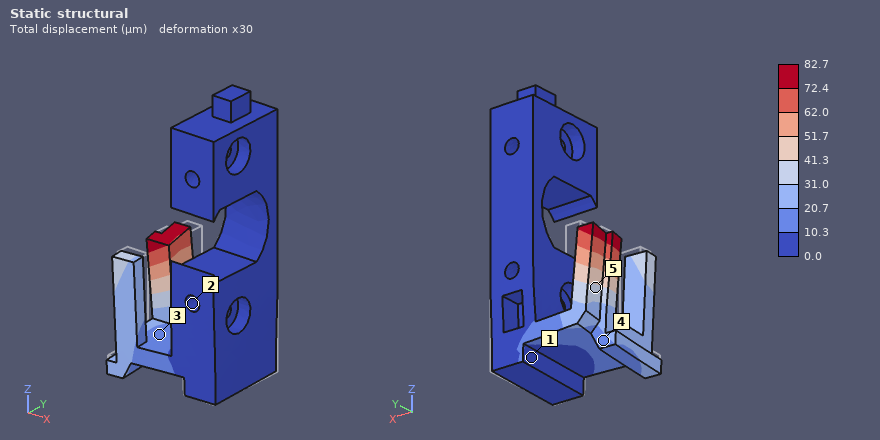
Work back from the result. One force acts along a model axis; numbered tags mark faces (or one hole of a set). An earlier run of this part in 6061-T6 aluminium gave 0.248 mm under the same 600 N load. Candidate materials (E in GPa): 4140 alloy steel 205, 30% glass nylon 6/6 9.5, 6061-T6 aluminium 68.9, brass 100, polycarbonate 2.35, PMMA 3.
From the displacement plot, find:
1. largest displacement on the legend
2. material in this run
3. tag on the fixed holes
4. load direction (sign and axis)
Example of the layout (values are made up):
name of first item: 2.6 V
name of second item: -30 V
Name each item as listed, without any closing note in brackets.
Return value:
largest displacement on the legend: 82.7 µm
material in this run: 4140 alloy steel
tag on the fixed holes: 2
load direction: -Y
